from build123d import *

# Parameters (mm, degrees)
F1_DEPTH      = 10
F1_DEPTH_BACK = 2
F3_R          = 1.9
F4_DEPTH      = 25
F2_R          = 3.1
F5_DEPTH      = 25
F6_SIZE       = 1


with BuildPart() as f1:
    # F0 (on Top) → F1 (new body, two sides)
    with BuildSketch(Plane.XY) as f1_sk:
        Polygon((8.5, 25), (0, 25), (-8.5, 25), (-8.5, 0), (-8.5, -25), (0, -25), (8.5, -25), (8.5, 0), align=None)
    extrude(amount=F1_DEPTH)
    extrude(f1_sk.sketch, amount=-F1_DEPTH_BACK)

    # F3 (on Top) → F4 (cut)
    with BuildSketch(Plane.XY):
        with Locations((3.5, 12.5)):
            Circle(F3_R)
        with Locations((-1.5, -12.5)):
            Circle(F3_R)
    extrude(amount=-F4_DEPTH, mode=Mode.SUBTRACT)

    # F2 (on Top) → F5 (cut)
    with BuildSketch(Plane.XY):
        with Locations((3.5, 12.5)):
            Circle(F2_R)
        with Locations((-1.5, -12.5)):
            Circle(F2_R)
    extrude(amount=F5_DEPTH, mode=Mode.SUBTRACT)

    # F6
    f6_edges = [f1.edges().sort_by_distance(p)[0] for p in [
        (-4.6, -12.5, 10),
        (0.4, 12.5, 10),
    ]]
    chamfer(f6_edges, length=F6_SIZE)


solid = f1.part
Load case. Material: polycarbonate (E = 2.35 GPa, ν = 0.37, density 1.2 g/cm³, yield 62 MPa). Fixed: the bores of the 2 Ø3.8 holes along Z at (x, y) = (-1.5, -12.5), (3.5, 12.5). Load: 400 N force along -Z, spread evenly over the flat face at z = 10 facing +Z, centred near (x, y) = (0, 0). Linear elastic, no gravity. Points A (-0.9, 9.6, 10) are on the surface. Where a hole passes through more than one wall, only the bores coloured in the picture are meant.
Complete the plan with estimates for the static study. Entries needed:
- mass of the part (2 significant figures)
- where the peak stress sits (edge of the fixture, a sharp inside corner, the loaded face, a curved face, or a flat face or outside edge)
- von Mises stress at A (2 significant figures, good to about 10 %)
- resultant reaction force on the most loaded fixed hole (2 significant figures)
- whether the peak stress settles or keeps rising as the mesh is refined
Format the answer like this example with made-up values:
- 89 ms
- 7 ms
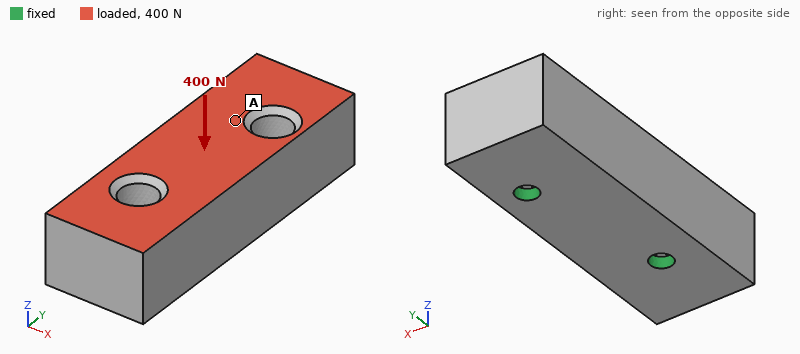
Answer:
- 11 g
- edge of the fixture
- 2.2 MPa
- 200 N
- keeps rising
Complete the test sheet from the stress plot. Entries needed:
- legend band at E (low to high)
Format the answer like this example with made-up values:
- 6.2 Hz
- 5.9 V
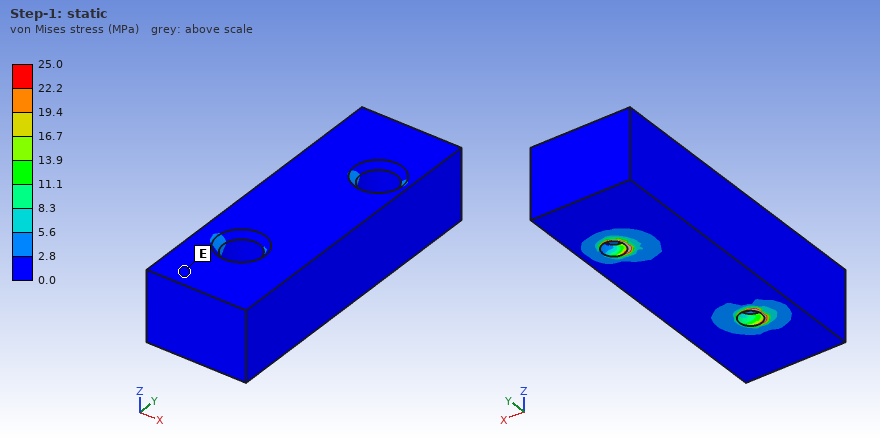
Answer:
- 0.0 to 2.8 MPa
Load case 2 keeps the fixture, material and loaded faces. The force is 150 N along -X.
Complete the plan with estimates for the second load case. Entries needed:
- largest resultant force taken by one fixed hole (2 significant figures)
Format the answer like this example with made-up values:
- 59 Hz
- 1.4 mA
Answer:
- 76 N
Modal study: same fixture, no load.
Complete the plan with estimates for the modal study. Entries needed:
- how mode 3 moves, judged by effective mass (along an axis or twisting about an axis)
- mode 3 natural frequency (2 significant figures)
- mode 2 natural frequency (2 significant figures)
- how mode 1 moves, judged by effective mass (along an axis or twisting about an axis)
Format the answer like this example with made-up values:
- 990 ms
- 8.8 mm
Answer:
- along Y
- 4600 Hz
- 4100 Hz
- along X
